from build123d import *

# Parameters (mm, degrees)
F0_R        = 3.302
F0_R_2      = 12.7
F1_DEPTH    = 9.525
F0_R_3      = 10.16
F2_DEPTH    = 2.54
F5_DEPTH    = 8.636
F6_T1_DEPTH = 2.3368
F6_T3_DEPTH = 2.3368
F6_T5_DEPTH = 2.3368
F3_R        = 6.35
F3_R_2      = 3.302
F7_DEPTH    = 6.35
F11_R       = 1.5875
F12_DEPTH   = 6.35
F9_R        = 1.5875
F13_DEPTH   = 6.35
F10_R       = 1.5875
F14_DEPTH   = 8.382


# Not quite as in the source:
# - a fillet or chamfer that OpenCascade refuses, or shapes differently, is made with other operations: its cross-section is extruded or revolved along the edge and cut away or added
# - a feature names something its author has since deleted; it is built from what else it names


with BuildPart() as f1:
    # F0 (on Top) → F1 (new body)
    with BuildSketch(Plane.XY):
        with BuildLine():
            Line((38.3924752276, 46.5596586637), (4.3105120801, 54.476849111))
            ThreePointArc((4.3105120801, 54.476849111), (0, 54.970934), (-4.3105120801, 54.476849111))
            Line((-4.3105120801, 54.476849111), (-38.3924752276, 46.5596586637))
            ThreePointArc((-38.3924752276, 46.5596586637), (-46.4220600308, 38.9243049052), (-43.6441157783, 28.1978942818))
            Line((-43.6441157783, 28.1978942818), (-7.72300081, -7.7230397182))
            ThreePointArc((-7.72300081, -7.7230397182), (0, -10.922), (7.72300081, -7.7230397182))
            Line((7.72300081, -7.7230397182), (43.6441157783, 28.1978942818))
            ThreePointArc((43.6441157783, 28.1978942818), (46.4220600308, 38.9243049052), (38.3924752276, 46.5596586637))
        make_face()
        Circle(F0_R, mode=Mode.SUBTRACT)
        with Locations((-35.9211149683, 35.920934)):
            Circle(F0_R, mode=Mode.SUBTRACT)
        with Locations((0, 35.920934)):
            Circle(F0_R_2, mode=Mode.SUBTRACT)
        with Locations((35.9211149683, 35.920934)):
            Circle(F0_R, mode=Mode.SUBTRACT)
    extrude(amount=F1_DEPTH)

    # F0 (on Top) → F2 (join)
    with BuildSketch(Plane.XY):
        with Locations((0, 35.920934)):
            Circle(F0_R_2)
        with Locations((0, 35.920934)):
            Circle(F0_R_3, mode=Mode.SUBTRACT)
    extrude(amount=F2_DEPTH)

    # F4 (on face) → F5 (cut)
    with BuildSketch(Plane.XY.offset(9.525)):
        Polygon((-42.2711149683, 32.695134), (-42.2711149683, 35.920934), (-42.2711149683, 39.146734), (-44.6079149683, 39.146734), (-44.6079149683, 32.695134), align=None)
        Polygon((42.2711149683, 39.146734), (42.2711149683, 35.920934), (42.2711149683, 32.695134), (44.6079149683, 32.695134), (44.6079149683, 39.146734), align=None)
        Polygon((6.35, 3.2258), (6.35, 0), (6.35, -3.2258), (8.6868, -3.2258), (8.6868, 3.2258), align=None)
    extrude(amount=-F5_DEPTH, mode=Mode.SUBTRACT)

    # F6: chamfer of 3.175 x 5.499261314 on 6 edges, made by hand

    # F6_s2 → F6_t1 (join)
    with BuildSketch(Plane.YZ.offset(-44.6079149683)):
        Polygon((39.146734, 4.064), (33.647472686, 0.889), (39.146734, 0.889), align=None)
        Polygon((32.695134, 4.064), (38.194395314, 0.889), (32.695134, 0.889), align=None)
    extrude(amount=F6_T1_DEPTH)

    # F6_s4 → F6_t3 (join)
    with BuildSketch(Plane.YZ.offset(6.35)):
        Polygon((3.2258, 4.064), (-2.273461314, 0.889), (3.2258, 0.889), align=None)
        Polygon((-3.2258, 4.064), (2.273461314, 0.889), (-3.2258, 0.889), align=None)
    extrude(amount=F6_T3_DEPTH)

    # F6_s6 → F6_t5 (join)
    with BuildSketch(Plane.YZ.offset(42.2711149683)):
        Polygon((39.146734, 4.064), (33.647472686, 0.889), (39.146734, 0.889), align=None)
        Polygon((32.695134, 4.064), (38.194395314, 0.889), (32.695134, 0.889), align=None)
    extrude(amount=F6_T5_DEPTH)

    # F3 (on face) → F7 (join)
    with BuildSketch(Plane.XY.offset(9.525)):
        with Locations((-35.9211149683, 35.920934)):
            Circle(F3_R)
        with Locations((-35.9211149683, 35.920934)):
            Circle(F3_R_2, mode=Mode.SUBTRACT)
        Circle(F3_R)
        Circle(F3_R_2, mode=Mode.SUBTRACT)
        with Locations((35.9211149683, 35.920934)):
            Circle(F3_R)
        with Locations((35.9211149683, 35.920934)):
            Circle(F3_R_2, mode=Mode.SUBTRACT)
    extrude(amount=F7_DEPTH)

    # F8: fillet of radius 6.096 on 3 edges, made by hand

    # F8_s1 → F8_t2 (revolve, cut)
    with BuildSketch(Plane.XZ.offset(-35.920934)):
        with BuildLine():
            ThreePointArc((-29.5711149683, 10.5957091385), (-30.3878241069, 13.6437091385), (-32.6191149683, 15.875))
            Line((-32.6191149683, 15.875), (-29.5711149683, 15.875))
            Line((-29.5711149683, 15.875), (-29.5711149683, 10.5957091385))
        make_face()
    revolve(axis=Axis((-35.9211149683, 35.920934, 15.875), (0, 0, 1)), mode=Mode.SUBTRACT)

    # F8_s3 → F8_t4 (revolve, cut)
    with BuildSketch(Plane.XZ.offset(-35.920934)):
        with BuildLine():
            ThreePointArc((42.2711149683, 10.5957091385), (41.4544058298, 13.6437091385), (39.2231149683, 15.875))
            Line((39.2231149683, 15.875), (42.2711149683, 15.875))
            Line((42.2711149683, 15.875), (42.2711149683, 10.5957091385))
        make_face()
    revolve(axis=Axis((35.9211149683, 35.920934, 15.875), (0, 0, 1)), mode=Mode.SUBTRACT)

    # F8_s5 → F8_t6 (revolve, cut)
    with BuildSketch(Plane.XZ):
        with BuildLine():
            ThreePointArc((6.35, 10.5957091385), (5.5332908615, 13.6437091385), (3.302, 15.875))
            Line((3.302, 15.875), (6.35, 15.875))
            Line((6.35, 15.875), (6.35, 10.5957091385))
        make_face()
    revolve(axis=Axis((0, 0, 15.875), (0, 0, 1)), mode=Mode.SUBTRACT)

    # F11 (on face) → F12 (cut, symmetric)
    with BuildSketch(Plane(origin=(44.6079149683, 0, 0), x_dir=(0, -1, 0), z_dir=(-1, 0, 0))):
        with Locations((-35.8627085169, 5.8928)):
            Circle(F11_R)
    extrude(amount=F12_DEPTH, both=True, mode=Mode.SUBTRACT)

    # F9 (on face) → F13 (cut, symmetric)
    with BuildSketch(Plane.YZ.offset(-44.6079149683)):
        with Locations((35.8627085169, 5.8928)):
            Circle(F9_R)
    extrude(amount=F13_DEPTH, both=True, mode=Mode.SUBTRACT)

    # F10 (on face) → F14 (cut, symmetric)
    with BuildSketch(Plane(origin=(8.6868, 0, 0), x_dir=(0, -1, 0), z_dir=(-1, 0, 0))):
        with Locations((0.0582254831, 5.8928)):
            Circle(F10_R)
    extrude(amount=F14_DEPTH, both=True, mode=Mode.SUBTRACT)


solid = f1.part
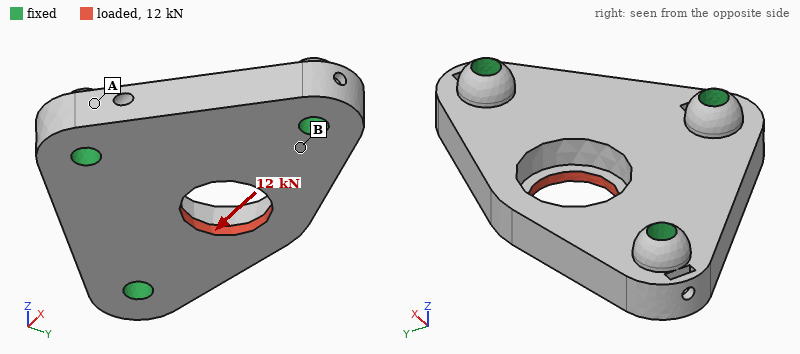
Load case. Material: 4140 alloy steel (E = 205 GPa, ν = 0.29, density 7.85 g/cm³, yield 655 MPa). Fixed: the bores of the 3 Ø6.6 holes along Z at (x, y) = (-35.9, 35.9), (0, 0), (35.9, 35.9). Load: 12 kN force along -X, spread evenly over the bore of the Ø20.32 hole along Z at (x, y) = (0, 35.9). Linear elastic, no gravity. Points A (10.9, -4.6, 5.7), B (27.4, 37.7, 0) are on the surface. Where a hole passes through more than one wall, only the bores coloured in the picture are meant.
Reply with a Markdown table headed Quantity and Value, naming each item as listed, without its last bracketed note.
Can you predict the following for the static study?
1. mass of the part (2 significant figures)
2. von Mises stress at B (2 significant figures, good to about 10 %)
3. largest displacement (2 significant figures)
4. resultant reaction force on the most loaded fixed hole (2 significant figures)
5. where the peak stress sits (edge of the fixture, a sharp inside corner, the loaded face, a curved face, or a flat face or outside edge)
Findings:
| Quantity | Value |
|---|---|
| mass of the part | 250 g |
| von Mises stress at B | 39 MPa |
| largest displacement | 7.6 µm |
| resultant reaction force on the most loaded fixed hole | 5.2 kN |
| where the peak stress sits | a sharp inside corner |
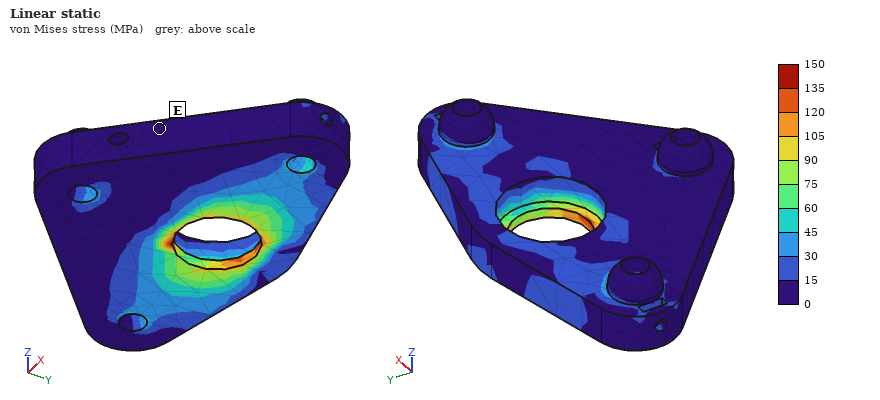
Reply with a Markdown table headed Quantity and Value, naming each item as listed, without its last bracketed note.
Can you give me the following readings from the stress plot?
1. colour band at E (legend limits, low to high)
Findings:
| Quantity | Value |
|---|---|
| colour band at E | 0 to 15 MPa |
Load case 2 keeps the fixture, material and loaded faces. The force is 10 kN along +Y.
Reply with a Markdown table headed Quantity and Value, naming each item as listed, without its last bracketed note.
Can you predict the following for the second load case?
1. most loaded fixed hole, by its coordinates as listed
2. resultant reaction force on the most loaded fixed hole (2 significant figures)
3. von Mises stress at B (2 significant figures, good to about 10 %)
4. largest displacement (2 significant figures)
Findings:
| Quantity | Value |
|---|---|
| most loaded fixed hole, by its coordinates as listed | (0, 0) |
| resultant reaction force on the most loaded fixed hole | 5.2 kN |
| von Mises stress at B | 36 MPa |
| largest displacement | 18 µm |
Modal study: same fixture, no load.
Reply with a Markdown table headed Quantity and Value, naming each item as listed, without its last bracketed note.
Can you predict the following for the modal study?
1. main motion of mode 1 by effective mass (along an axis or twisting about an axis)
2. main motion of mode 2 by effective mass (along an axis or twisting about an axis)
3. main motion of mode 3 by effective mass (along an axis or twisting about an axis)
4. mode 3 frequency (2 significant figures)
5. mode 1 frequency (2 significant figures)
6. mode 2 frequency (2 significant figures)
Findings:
| Quantity | Value |
|---|---|
| main motion of mode 1 by effective mass | along Z |
| main motion of mode 2 by effective mass | along Z |
| main motion of mode 3 by effective mass | twisting about Y |
| mode 3 frequency | 18 kHz |
| mode 1 frequency | 10000 Hz |
| mode 2 frequency | 17 kHz |
